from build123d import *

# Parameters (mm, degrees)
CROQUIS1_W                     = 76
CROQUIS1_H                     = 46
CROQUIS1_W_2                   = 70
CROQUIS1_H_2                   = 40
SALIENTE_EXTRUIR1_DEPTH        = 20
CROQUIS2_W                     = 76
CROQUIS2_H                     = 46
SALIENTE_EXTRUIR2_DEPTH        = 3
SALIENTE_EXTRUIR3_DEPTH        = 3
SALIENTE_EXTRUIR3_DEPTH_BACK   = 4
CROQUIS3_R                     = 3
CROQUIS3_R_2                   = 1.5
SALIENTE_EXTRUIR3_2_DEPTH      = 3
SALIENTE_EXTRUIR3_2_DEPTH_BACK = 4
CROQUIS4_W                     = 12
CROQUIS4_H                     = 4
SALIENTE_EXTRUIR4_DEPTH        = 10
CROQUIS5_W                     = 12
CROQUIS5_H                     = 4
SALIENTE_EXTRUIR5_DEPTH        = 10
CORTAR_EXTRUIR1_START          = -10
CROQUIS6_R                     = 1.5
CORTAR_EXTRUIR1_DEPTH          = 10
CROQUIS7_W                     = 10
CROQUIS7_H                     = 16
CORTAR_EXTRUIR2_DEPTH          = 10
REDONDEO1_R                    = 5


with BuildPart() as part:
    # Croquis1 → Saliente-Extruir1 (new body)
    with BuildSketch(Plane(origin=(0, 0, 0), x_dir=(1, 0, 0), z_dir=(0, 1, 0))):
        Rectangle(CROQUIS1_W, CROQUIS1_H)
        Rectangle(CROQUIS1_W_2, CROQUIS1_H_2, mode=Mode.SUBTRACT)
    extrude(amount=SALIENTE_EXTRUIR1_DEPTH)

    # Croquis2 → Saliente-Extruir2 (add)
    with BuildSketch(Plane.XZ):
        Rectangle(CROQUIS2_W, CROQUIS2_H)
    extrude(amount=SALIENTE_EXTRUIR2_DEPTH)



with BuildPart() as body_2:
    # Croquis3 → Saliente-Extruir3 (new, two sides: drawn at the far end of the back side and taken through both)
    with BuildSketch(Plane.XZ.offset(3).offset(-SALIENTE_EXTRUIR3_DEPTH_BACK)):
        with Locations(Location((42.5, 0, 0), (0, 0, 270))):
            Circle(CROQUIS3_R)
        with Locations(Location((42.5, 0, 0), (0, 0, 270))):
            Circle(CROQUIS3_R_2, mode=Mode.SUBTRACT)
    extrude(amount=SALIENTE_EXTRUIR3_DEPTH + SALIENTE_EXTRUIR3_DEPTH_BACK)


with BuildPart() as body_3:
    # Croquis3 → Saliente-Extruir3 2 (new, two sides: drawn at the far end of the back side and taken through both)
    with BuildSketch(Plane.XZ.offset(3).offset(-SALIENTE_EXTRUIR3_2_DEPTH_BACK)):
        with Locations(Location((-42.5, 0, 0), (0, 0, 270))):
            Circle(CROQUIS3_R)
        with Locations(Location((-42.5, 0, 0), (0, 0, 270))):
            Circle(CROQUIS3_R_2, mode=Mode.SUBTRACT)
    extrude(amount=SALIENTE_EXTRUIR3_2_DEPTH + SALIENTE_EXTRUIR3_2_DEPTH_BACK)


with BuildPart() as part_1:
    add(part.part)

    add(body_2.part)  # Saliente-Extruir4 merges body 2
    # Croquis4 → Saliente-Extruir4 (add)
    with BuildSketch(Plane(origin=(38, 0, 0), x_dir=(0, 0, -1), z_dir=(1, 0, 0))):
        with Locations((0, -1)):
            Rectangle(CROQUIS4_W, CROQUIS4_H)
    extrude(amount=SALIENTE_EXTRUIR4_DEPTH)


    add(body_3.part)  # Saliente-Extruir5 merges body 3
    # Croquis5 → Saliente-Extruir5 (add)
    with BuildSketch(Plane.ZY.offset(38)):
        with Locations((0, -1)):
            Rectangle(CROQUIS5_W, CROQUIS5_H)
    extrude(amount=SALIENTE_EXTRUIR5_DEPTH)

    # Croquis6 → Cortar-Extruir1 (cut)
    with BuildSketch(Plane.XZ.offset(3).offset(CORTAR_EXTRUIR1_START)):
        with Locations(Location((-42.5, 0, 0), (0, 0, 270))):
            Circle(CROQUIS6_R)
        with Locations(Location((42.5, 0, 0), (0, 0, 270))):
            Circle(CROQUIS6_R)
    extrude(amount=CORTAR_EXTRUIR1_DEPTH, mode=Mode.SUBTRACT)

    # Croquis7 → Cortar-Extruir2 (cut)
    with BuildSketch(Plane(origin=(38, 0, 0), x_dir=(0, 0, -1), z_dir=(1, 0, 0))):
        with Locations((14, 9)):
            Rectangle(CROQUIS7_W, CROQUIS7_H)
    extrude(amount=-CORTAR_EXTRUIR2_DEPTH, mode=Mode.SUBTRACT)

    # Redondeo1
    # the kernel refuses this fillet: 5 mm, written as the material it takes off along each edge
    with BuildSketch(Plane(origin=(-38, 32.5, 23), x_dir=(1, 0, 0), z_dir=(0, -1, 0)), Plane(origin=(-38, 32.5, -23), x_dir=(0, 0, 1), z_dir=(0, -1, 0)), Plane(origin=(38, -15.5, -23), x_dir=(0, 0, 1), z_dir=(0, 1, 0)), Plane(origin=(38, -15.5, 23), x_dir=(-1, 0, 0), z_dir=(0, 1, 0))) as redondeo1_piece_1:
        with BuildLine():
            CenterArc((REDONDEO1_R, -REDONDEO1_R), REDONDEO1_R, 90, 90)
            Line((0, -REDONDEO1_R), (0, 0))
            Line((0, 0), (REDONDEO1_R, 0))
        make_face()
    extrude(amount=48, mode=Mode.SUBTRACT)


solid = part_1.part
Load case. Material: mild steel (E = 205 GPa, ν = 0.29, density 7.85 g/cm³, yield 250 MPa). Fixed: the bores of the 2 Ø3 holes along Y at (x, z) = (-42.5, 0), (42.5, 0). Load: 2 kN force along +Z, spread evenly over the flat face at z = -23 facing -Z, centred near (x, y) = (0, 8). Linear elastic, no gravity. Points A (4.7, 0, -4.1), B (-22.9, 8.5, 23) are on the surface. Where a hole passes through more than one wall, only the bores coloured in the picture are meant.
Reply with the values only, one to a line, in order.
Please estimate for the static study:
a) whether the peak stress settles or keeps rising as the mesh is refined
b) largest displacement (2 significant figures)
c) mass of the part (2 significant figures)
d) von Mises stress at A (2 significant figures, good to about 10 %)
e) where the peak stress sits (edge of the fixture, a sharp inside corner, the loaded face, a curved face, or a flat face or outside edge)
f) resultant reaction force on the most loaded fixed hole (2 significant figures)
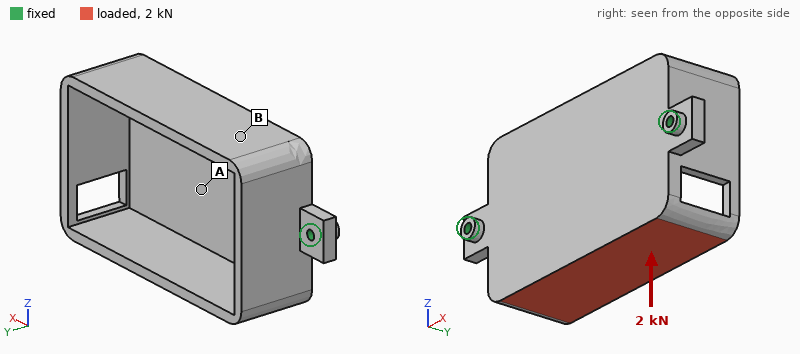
keeps rising
0.18 mm
190 g
37 MPa
edge of the fixture
1.0 kN
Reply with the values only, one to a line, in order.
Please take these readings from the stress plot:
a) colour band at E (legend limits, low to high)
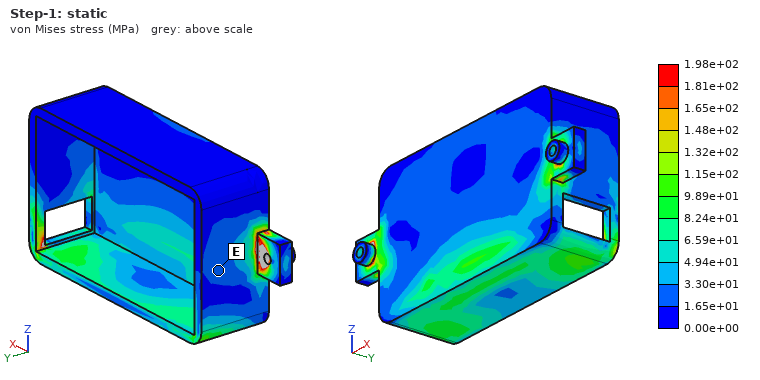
1.65e+01 to 3.30e+01 MPa
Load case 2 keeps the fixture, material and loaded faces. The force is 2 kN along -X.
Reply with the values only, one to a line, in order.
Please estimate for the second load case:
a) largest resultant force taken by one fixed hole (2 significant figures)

1.2 kN
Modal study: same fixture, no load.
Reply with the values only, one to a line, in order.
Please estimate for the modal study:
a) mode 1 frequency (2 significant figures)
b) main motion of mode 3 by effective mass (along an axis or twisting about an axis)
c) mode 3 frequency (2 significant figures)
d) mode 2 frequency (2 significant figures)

1700 Hz
along Y
4000 Hz
3200 Hz
